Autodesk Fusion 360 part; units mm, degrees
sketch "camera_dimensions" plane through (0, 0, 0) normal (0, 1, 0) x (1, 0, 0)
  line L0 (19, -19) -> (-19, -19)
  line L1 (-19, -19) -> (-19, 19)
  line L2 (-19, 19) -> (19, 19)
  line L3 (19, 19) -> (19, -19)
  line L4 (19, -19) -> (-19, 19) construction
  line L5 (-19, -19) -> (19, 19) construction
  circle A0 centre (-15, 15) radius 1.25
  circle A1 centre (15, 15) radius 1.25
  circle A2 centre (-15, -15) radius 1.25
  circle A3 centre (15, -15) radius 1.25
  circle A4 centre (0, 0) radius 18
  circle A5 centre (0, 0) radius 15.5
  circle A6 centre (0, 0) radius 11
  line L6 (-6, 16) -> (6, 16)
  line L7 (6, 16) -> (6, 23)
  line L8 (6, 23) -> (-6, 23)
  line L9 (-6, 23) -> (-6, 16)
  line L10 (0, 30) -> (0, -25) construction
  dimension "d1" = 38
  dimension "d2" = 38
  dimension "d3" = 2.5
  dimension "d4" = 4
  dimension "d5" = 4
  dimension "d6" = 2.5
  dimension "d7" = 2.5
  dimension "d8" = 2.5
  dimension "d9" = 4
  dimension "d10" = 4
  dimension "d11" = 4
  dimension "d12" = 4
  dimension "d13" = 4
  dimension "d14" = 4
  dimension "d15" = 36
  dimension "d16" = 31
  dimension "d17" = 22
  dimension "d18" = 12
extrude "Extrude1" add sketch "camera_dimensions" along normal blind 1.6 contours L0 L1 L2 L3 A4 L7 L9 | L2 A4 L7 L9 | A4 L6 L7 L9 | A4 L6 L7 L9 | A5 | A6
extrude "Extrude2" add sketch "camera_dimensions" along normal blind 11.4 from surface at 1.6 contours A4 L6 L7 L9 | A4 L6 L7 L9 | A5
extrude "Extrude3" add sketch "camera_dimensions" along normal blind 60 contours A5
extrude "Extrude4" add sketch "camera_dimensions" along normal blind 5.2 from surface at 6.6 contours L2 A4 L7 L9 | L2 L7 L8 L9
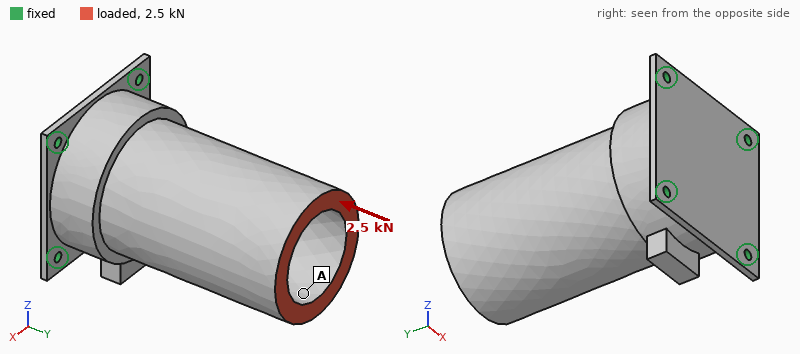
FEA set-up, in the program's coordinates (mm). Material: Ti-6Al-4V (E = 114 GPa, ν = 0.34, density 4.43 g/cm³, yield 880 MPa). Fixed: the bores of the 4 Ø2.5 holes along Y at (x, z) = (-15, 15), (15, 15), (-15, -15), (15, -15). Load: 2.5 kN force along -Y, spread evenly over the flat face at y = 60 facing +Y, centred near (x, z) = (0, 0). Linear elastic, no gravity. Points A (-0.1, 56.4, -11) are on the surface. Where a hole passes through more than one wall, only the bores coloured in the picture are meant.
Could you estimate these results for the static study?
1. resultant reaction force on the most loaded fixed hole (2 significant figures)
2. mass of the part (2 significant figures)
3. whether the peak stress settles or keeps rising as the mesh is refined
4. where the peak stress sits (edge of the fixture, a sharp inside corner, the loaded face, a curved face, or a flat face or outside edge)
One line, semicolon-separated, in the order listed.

700 N; 120 g; keeps rising; edge of the fixture
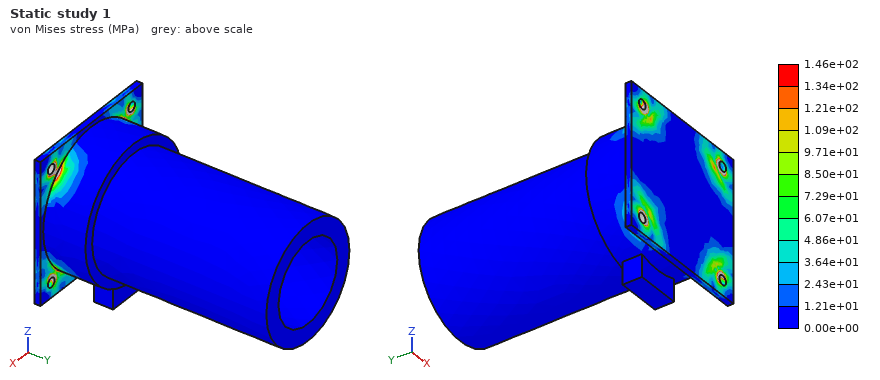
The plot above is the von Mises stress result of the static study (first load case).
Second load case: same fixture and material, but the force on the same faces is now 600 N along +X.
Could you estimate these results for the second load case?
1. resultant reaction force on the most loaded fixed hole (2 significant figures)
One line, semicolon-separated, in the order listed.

710 N
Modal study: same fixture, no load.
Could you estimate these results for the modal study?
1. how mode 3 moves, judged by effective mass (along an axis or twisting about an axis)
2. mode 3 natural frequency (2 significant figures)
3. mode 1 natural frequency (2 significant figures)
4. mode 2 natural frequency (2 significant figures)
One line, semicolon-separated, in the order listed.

along Y; 6500 Hz; 2600 Hz; 2600 Hz
